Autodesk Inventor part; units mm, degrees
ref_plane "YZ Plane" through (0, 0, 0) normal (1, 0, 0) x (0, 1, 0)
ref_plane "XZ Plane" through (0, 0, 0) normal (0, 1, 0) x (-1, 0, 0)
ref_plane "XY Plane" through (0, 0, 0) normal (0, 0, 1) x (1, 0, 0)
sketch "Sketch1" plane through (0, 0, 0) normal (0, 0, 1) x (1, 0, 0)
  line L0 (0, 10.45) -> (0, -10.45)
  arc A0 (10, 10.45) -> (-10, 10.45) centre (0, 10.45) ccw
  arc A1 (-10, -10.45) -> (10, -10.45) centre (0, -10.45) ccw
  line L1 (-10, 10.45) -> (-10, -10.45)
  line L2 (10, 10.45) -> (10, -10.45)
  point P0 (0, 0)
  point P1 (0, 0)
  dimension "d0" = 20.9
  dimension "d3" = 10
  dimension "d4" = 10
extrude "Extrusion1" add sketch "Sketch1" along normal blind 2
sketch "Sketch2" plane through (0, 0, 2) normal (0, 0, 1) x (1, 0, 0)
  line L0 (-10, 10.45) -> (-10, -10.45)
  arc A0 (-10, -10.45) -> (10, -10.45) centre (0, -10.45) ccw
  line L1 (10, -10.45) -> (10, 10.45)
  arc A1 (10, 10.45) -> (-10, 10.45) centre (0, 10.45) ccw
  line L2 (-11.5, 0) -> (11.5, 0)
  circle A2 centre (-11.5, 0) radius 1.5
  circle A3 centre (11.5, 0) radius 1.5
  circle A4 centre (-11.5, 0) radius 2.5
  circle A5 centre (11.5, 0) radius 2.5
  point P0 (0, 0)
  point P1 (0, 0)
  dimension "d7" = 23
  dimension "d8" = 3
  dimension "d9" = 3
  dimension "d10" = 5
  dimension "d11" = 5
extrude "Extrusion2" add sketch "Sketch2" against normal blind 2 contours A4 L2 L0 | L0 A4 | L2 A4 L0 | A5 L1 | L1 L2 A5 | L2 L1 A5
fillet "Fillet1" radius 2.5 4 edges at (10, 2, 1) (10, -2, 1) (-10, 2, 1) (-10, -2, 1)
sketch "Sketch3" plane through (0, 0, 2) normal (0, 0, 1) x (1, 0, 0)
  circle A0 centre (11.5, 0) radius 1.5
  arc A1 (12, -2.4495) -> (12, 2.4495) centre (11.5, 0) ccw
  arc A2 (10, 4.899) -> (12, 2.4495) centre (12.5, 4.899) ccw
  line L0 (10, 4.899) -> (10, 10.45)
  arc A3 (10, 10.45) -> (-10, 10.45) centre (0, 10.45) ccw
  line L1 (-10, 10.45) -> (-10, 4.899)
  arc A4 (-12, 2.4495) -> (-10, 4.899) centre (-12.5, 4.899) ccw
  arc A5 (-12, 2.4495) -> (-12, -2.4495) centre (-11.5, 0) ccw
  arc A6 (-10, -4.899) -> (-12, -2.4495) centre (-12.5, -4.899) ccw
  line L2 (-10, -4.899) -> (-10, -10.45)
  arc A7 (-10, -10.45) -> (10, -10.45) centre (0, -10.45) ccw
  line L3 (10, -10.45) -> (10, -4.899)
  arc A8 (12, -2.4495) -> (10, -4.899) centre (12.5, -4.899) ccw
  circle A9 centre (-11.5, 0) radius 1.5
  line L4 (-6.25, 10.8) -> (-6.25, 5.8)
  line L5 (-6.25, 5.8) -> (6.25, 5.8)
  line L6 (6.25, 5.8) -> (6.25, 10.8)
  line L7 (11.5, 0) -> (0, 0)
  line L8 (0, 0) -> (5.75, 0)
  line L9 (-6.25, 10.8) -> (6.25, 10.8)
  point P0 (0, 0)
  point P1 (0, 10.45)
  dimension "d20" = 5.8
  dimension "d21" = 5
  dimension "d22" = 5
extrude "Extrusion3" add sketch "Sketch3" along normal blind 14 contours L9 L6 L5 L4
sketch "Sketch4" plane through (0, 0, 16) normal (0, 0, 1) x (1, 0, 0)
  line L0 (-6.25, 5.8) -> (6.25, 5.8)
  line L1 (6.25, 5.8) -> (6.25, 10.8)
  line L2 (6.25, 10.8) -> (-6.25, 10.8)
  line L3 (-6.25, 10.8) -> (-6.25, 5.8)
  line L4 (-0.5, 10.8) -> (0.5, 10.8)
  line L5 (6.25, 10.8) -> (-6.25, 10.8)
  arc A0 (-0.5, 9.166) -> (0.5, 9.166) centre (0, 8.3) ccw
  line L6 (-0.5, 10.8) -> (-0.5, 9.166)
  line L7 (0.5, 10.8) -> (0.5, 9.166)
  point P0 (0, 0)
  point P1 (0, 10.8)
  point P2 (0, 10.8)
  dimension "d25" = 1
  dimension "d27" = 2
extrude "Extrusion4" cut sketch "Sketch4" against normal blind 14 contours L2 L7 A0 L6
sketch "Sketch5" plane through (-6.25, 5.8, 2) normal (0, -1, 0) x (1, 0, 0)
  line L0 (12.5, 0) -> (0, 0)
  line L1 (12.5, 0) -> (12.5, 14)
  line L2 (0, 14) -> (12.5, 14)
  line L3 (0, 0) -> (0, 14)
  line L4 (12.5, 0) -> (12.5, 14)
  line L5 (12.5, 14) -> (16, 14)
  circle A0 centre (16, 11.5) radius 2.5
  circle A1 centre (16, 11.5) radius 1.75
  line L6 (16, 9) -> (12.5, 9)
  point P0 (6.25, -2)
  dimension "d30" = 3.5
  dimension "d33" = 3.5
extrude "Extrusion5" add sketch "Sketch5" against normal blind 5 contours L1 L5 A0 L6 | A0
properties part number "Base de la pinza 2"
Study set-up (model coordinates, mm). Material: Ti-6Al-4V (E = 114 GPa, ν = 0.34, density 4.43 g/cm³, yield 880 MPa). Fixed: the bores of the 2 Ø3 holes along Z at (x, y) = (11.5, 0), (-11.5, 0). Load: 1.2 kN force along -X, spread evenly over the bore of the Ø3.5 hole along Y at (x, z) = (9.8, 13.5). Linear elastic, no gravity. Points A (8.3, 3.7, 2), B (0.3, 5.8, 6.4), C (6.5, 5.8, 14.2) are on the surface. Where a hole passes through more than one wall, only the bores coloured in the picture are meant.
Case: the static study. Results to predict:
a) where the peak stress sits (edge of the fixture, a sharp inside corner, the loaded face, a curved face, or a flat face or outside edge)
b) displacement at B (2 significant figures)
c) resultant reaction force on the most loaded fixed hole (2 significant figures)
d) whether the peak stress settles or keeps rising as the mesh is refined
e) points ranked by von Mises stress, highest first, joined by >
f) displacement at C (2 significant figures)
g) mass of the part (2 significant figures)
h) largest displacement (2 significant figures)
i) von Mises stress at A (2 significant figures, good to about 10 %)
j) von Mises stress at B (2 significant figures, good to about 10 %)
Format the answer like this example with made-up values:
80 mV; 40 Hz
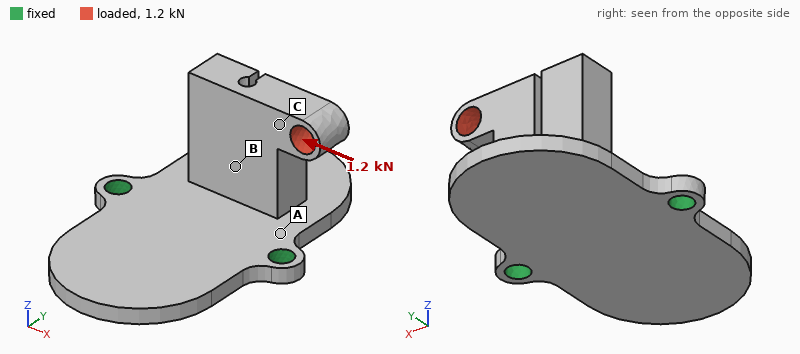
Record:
edge of the fixture; 0.077 mm; 1.1 kN; keeps rising; A > B > C; 0.21 mm; 11 g; 0.26 mm; 350 MPa; 120 MPa
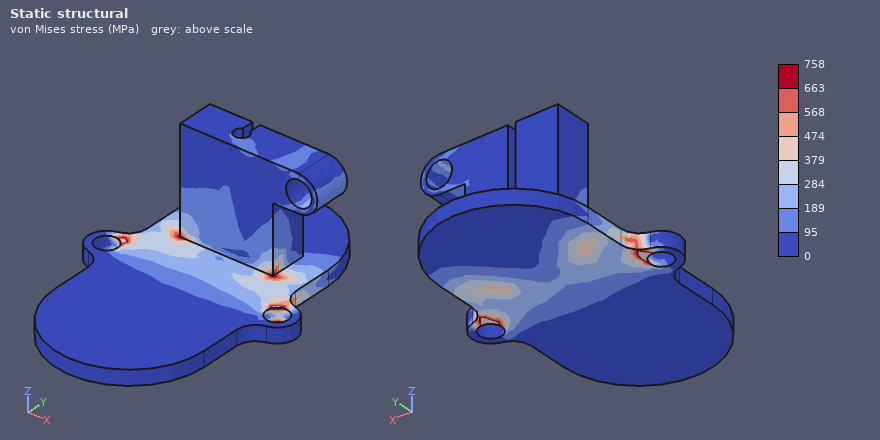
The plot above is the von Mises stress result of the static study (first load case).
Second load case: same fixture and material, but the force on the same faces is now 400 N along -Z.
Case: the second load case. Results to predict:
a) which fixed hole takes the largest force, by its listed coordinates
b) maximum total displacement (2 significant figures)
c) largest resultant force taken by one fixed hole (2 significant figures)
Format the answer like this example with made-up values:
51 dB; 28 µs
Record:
(11.5, 0); 0.24 mm; 420 N
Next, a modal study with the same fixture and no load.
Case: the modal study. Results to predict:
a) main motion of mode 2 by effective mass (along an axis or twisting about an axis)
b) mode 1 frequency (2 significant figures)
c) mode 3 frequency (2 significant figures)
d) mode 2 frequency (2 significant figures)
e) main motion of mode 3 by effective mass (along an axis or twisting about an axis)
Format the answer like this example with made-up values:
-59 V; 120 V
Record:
along Z; 2500 Hz; 7500 Hz; 4300 Hz; along X
